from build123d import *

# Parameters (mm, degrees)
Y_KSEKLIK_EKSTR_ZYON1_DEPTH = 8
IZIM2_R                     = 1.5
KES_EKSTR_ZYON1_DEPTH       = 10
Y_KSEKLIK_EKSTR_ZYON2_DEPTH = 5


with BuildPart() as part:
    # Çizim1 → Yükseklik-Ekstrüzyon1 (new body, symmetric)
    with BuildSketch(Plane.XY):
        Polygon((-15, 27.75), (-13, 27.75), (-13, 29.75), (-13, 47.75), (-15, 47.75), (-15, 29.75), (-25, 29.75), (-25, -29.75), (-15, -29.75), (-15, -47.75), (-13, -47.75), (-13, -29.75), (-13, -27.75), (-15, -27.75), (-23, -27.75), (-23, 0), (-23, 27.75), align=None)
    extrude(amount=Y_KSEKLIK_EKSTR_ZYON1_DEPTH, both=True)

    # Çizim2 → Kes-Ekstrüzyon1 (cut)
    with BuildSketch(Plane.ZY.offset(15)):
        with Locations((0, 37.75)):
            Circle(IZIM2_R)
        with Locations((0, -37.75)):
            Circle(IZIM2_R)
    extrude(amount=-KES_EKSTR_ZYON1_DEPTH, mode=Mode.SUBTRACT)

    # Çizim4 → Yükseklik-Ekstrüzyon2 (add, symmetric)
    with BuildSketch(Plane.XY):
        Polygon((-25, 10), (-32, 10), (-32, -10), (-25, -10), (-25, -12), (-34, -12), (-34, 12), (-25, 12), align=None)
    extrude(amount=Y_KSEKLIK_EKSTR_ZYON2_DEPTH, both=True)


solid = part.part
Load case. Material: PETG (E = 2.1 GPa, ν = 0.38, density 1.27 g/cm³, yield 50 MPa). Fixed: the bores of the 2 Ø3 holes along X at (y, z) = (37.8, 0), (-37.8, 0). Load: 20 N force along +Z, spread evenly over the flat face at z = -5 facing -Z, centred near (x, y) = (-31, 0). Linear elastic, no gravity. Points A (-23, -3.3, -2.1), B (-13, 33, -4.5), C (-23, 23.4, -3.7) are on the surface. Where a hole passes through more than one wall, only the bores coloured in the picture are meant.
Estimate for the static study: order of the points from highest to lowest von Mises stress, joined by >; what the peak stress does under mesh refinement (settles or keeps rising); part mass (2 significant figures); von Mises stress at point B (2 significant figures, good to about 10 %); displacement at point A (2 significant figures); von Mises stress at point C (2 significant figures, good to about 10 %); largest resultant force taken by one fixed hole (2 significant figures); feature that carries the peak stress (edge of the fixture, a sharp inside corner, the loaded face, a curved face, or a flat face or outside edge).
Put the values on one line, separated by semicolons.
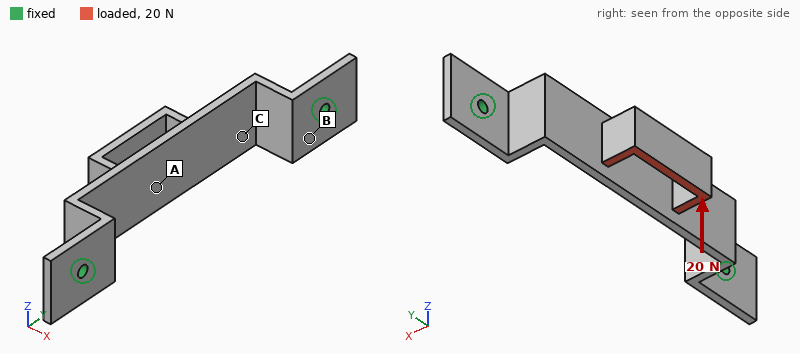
B > C > A; keeps rising; 5.6 g; 6.4 MPa; 0.37 mm; 4.2 MPa; 10 N; edge of the fixture
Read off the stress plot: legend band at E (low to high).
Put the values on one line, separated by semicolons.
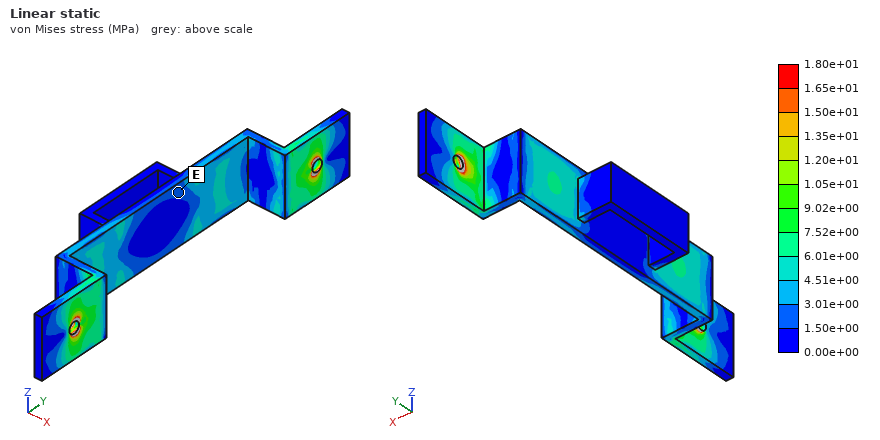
1.50e+00 to 3.01e+00 MPa
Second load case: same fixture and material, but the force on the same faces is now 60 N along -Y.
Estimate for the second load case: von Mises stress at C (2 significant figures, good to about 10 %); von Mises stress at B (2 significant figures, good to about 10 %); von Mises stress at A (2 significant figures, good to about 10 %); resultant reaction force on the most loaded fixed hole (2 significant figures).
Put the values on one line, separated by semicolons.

8.7 MPa; 7.4 MPa; 3.3 MPa; 33 N
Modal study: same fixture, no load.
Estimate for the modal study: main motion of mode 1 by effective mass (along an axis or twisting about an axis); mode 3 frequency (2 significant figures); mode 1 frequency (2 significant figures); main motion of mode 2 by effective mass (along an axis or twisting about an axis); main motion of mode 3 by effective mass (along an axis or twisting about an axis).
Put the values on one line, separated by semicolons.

along Z; 780 Hz; 560 Hz; along X; along Y
